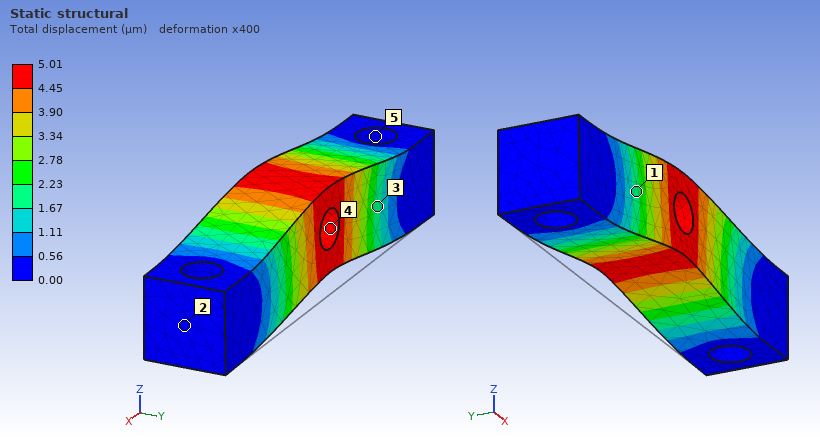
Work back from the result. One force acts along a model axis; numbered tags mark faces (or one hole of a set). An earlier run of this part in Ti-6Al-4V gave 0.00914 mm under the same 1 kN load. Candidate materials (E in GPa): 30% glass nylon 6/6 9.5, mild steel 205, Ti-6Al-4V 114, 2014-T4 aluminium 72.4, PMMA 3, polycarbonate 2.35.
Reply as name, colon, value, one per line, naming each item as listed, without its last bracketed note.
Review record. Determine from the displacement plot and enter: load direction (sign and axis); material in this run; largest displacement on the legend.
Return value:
load direction: +Z
material in this run: mild steel
largest displacement on the legend: 5.01 µm
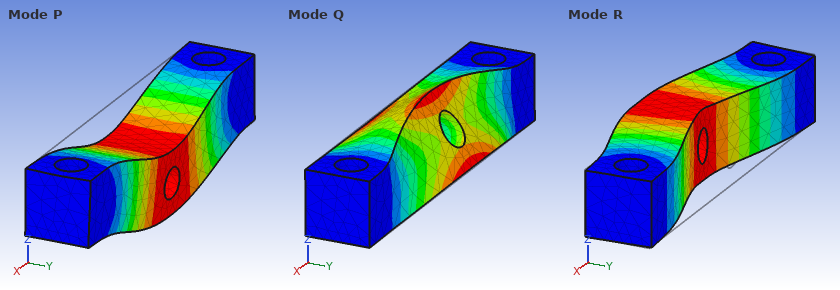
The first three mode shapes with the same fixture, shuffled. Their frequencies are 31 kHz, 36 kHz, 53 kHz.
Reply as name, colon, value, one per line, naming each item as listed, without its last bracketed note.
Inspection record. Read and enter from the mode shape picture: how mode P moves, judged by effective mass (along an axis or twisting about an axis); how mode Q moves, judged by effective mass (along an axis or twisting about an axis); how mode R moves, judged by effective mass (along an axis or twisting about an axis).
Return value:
how mode P moves, judged by effective mass: along Z
how mode Q moves, judged by effective mass: twisting about X
how mode R moves, judged by effective mass: along Y
